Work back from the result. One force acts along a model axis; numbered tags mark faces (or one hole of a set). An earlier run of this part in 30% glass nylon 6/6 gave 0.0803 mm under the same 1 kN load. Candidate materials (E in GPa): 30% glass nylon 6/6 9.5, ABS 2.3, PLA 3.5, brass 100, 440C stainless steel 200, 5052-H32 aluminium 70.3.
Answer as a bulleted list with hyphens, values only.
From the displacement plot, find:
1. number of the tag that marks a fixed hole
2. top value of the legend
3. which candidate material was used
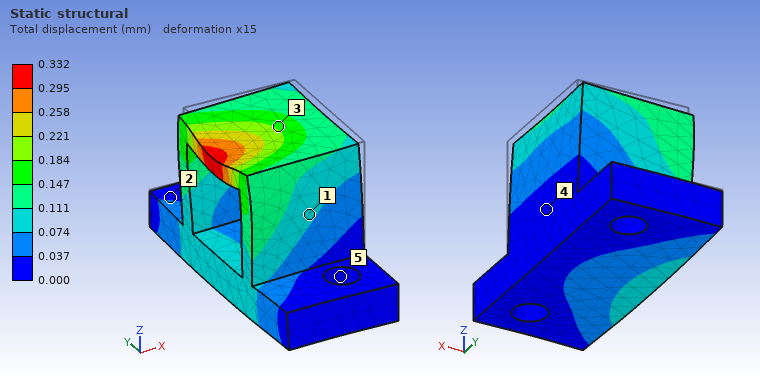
- 5
- 0.332 mm
- ABS
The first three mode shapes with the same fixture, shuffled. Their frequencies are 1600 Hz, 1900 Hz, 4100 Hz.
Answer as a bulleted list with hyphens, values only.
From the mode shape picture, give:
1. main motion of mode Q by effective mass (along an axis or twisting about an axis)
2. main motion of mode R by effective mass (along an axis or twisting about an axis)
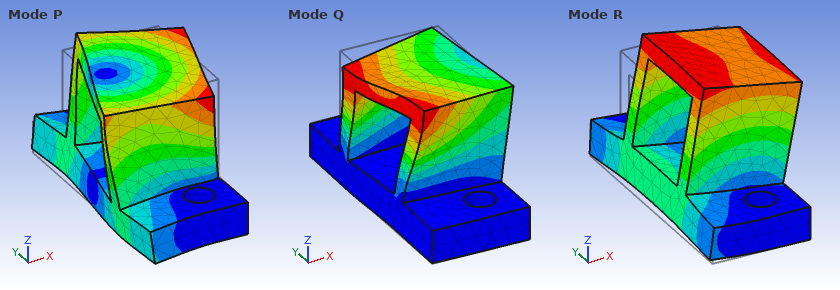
- along Y
- along X
